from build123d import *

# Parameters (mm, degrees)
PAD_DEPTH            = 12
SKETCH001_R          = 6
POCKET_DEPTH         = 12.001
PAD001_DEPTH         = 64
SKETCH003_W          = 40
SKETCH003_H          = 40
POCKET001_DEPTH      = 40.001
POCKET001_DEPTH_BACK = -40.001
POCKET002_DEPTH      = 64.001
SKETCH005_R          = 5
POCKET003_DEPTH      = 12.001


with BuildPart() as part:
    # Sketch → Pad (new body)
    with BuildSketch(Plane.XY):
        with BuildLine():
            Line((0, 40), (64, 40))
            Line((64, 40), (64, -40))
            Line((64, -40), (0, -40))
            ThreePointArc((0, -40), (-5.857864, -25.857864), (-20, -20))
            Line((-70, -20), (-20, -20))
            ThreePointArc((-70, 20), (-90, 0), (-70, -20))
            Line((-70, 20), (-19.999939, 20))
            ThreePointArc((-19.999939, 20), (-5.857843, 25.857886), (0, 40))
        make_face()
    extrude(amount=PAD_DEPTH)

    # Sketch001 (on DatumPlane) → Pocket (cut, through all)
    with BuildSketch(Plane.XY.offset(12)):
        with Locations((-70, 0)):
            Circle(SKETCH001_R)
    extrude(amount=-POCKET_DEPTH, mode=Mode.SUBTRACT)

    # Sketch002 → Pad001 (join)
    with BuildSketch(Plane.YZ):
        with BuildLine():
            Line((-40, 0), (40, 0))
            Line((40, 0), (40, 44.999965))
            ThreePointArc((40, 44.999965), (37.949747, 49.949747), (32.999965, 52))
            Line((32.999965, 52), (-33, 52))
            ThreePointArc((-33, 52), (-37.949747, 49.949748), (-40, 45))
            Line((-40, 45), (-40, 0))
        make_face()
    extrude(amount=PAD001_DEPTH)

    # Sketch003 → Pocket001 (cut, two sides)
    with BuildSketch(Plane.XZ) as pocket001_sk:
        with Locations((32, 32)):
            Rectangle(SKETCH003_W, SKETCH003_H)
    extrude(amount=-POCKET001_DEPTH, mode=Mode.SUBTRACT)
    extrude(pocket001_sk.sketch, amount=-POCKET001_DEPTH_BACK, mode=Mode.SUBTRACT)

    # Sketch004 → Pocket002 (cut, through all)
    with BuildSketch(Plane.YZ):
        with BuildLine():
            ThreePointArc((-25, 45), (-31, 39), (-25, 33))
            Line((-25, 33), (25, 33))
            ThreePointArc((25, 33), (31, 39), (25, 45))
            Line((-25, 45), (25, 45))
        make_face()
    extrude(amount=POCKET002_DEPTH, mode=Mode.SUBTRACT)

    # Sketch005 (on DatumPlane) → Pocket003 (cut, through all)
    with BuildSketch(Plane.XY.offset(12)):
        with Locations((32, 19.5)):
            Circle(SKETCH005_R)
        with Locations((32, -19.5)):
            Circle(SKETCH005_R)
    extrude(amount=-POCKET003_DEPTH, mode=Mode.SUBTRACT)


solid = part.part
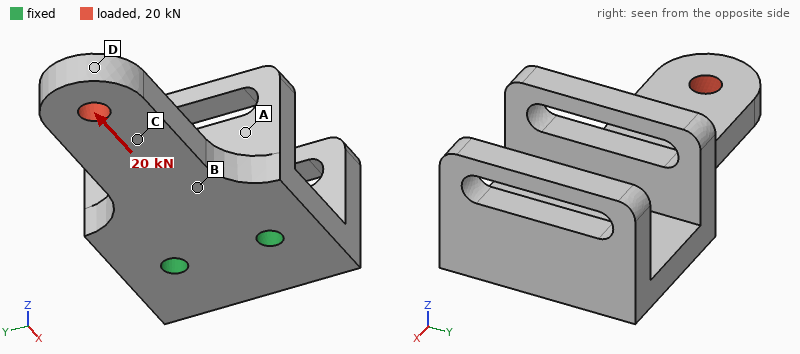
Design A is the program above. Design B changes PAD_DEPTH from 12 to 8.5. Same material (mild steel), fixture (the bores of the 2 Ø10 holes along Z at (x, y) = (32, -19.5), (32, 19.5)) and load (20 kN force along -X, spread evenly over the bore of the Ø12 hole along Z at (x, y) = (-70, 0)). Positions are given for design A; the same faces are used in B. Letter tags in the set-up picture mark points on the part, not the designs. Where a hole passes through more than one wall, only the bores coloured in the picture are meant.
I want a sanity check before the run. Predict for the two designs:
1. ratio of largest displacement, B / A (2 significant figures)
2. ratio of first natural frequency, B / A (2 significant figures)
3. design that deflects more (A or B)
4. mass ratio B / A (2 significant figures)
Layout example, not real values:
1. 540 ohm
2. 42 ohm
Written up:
1. 2.5
2. 0.88
3. B
4. 0.92
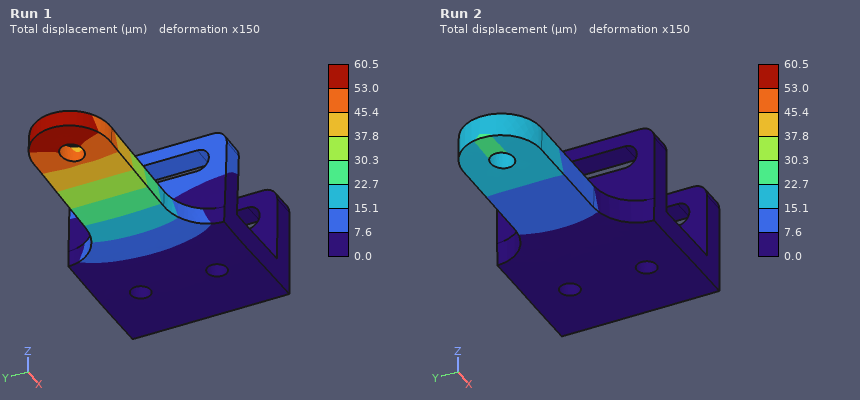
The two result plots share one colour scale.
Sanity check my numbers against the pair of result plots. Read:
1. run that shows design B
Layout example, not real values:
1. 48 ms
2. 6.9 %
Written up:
1. Run 1
